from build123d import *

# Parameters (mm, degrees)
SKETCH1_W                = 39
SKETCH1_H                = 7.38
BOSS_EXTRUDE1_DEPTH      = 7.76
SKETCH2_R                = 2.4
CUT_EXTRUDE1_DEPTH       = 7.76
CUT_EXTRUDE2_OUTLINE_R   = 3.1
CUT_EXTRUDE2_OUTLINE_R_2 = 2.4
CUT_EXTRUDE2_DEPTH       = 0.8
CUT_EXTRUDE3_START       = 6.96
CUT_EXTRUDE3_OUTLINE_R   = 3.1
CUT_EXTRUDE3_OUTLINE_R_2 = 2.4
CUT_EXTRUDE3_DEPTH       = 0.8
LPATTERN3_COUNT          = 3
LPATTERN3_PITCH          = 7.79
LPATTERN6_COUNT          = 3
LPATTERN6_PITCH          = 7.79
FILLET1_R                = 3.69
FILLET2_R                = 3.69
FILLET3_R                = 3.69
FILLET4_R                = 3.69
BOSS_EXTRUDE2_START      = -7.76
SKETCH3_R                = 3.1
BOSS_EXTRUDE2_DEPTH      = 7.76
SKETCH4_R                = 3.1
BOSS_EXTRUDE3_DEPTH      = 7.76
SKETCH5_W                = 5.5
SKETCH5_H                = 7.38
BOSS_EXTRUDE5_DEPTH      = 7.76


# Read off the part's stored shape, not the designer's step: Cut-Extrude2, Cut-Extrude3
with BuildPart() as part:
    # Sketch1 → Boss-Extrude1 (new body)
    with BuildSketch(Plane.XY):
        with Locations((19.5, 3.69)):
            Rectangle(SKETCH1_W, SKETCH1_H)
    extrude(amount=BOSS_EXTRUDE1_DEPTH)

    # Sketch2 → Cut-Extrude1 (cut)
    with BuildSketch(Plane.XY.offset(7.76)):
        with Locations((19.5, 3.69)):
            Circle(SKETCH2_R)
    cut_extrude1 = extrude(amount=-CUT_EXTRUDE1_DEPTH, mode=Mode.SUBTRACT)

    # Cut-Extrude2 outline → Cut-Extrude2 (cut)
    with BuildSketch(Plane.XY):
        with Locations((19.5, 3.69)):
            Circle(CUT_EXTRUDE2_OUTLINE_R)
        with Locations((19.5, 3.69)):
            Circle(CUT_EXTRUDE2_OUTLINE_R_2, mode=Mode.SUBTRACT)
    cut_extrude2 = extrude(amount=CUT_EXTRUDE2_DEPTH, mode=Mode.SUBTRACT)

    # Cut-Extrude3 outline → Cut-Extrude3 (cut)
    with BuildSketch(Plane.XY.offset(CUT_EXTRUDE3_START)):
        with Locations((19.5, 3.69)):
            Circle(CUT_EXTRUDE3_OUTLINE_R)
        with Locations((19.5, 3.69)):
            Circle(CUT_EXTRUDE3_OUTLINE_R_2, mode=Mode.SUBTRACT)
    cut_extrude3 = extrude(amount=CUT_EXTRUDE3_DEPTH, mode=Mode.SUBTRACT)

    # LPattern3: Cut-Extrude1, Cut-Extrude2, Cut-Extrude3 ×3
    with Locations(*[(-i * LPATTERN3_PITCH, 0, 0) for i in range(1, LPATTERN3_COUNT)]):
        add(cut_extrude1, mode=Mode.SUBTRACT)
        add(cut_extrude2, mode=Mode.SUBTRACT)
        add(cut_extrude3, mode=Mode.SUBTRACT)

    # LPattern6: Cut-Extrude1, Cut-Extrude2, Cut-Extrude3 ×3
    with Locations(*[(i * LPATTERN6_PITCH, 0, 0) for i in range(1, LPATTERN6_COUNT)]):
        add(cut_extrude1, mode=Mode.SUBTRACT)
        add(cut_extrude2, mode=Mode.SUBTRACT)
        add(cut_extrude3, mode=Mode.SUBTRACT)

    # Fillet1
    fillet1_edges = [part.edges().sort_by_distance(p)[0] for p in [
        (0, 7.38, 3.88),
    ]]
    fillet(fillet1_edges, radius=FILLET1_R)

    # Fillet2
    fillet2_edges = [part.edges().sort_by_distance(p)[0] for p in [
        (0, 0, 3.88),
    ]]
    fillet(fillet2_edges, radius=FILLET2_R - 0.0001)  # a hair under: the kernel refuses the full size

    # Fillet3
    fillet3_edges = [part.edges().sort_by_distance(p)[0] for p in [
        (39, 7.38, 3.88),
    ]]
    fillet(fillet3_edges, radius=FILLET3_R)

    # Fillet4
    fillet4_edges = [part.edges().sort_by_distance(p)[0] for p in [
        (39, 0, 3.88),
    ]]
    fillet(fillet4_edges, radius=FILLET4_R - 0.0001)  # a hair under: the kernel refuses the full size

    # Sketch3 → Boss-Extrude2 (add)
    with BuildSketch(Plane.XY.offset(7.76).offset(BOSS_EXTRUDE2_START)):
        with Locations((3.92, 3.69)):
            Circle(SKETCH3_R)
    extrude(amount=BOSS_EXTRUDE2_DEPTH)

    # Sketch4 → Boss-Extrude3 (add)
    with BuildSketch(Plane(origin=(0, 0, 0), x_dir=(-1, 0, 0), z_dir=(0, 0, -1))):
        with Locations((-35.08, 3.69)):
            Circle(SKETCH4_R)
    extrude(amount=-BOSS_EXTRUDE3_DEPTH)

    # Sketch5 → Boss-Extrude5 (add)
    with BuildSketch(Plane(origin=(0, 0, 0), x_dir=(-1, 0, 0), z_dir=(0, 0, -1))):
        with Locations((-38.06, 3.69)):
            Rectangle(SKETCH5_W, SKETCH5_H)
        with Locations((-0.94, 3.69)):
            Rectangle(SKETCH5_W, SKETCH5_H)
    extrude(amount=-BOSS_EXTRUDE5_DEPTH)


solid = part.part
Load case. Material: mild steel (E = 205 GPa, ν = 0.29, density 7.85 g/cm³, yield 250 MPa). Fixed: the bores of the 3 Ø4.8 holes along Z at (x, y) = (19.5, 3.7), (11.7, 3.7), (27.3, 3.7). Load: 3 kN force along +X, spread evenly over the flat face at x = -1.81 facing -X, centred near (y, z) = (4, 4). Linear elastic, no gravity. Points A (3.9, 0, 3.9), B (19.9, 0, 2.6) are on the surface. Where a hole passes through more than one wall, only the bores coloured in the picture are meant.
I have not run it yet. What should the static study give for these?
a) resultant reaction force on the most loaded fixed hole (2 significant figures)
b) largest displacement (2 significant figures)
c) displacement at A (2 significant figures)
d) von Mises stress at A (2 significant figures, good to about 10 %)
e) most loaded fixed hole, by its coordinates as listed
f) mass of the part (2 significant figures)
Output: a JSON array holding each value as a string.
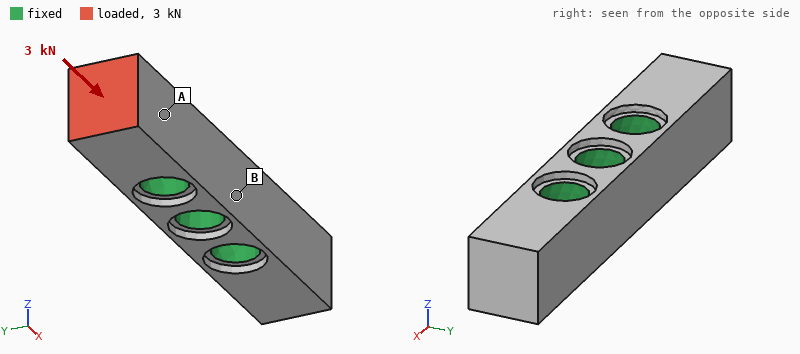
["2.9 kN", "3.2 µm", "1.7 µm", "54 MPa", "(11.7, 3.7)", "15 g"]
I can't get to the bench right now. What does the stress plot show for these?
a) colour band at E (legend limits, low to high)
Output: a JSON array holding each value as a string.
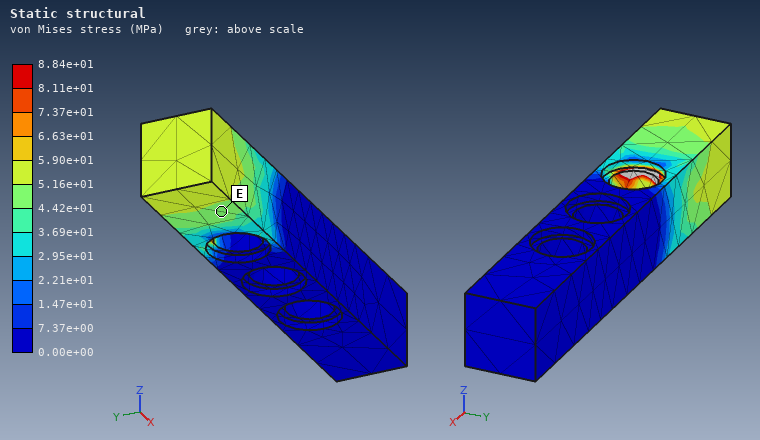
["4.42e+01 to 5.16e+01 MPa"]
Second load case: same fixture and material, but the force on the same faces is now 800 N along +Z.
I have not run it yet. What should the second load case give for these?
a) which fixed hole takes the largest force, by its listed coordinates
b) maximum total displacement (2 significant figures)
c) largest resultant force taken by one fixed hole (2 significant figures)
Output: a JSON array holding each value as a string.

["(11.7, 3.7)", "14 µm", "840 N"]
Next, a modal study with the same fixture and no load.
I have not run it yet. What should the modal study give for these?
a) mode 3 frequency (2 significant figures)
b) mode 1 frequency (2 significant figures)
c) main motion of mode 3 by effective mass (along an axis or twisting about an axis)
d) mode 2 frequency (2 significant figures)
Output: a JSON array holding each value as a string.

["31 kHz", "30 kHz", "along Z", "30 kHz"]
